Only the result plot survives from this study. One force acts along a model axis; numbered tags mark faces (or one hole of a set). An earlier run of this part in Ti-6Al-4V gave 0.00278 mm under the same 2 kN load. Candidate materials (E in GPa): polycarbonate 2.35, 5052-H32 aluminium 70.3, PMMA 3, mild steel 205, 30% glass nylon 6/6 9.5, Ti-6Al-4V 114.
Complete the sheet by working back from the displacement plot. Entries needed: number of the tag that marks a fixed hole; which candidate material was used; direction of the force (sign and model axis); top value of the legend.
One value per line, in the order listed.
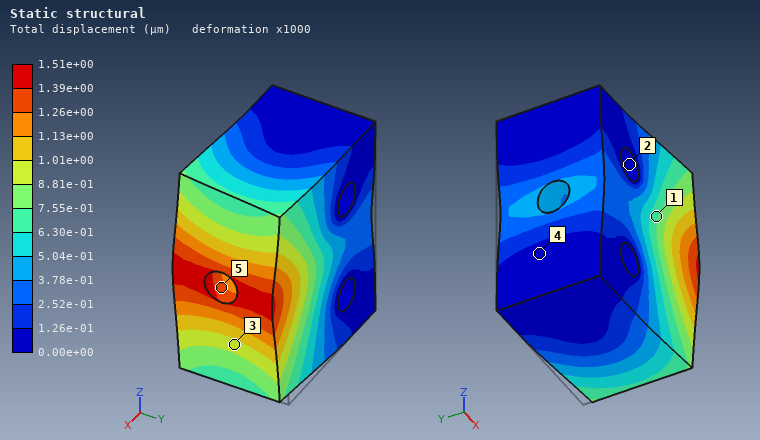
2
mild steel
-Y
1.51e+00 µm
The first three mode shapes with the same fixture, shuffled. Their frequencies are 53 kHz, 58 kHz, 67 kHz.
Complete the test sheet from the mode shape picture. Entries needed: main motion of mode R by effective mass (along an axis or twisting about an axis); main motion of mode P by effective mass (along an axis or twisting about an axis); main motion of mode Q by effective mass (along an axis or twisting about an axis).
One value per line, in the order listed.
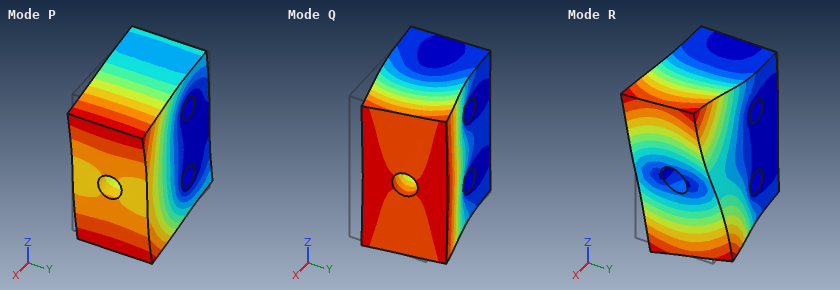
twisting about X
along Z
along Y
